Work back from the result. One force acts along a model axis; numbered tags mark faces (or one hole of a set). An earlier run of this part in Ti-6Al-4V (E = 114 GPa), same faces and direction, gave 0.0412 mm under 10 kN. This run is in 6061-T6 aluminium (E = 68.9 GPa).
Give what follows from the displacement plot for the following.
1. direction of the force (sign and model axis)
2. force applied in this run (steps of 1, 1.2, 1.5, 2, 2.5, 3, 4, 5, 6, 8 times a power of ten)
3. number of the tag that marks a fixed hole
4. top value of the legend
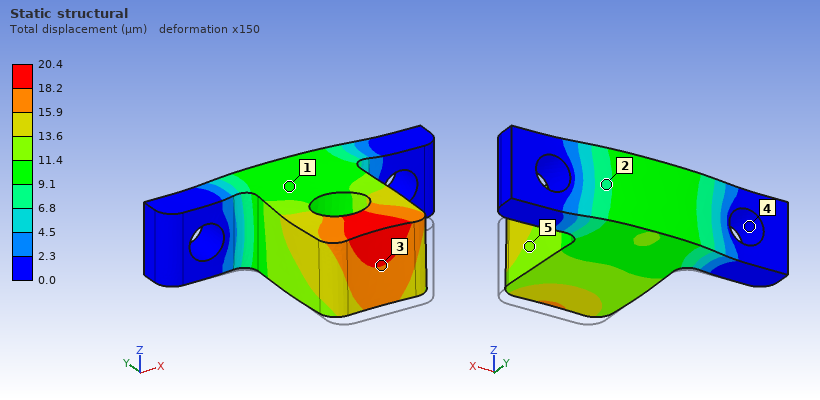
+Y
3 kN
4
20.4 µm
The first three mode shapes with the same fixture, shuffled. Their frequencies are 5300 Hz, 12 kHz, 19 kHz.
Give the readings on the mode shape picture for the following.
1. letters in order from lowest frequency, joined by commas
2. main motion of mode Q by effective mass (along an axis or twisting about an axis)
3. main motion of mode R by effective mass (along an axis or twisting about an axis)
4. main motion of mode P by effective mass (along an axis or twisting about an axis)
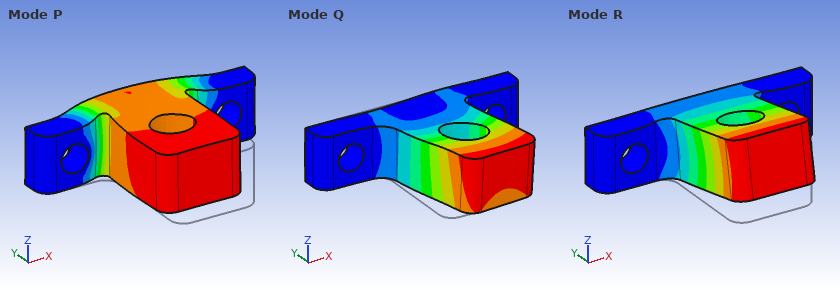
R, Q, P
along X
along Z
along Y
